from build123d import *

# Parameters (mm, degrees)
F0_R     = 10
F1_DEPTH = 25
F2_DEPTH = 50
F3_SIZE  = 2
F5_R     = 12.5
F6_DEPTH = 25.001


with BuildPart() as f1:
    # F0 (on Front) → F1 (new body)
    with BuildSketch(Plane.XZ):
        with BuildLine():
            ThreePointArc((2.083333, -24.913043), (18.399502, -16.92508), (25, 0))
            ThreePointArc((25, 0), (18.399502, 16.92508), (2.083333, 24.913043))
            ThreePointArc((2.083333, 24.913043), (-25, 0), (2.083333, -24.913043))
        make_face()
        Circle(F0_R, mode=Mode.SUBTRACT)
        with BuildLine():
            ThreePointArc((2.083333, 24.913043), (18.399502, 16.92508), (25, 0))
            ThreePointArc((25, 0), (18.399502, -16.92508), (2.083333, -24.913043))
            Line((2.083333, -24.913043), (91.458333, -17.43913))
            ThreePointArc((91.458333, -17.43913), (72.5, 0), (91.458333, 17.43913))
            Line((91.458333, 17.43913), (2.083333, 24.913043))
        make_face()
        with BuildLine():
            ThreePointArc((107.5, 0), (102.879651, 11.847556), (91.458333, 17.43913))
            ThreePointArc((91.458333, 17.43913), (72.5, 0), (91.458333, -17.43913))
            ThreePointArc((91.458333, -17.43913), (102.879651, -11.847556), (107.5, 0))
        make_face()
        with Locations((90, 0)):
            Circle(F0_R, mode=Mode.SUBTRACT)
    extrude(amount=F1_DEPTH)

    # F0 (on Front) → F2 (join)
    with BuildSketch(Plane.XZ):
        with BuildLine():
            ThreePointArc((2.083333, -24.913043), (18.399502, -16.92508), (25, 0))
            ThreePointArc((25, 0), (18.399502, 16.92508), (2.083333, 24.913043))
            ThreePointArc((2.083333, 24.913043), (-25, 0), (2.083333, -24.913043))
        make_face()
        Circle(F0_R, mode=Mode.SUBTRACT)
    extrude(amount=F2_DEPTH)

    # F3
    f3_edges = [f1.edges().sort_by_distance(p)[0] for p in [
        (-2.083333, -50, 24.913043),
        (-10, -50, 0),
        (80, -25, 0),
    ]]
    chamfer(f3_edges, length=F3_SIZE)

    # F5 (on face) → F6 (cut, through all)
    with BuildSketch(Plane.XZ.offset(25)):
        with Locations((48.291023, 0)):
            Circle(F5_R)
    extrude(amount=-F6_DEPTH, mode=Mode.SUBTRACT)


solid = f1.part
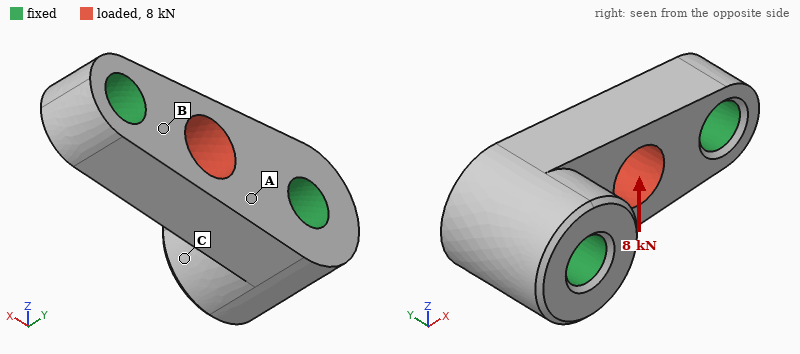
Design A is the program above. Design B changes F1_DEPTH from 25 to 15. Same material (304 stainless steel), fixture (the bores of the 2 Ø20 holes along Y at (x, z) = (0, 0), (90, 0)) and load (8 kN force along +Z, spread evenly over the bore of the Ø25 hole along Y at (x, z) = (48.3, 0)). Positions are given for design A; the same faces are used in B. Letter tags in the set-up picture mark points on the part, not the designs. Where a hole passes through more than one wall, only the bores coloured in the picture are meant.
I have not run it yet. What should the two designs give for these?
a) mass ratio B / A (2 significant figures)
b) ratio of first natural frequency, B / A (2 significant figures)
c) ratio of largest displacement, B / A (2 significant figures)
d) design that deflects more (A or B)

0.83
0.81
1.6
B
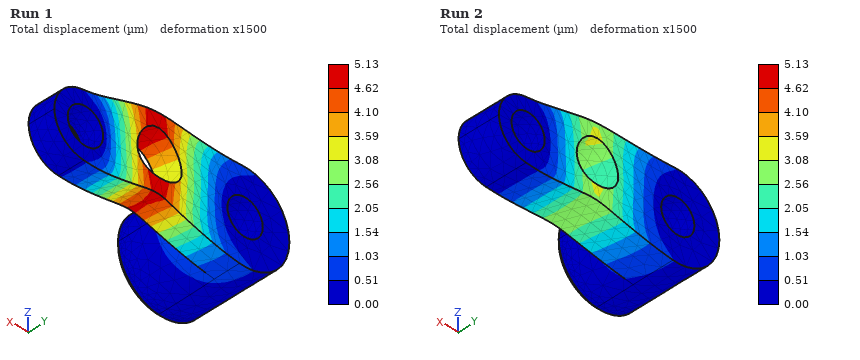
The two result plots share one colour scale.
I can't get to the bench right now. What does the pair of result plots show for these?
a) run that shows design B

Run 1
